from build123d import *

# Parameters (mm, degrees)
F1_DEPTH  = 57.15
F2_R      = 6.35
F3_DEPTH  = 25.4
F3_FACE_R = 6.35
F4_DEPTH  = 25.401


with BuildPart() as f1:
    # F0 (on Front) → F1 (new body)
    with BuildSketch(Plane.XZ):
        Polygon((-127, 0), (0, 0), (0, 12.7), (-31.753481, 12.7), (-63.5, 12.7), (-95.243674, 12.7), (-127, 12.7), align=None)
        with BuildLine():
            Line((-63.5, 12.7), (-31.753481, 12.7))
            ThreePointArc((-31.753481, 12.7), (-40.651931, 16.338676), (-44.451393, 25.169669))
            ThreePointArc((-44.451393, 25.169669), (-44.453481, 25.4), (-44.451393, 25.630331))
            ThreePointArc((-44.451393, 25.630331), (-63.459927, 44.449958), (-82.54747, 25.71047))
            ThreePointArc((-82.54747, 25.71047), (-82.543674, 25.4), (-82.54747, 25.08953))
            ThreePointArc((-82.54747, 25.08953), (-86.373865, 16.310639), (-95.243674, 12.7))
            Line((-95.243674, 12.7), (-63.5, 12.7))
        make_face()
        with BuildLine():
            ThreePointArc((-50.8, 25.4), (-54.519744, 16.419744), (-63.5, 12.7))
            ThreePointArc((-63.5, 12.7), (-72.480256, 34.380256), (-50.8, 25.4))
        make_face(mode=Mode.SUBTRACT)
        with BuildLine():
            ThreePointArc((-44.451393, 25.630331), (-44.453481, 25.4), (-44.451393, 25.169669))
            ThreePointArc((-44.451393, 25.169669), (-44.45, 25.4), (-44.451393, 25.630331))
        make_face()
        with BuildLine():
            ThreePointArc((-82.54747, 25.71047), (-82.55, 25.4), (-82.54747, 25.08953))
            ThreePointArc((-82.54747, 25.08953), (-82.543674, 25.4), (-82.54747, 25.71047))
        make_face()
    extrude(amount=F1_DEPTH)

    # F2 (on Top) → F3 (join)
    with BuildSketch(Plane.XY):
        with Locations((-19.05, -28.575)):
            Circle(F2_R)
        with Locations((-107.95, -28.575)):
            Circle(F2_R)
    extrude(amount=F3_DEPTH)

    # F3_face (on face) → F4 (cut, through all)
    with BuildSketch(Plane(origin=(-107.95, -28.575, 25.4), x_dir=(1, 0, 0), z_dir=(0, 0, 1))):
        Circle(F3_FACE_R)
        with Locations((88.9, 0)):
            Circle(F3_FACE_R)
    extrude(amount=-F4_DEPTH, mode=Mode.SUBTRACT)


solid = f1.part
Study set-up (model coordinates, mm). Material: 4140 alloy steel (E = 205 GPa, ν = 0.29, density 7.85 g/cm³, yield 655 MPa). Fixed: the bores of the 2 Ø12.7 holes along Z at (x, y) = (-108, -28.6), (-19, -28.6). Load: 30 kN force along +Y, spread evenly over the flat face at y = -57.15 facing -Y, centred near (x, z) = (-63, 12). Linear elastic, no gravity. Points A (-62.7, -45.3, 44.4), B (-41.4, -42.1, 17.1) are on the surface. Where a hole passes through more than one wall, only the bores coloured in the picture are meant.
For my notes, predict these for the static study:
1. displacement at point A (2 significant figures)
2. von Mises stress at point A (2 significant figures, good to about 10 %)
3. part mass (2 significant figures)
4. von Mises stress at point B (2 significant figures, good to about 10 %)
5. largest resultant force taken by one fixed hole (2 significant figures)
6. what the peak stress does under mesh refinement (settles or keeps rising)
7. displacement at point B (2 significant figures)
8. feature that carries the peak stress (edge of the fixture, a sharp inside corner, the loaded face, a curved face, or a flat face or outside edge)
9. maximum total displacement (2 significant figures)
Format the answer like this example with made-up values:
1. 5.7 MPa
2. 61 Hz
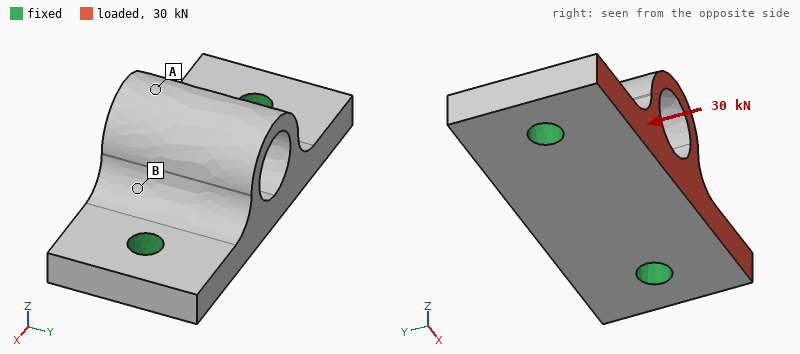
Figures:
1. 33 µm
2. 14 MPa
3. 970 g
4. 37 MPa
5. 15 kN
6. keeps rising
7. 14 µm
8. edge of the fixture
9. 37 µm
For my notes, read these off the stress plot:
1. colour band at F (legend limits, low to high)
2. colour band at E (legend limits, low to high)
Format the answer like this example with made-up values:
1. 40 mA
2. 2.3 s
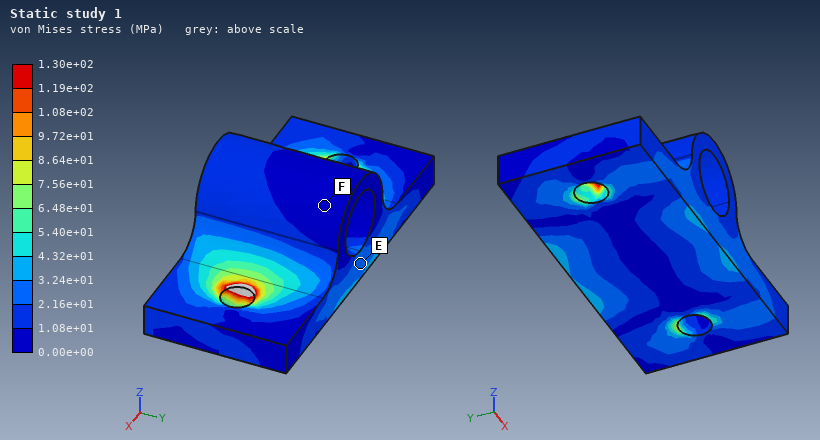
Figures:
1. 0.00e+00 to 1.08e+01 MPa
2. 2.16e+01 to 3.24e+01 MPa
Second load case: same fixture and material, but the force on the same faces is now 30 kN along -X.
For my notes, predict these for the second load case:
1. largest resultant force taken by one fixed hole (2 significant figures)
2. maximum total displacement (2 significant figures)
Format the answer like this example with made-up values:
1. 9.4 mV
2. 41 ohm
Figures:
1. 17 kN
2. 25 µm
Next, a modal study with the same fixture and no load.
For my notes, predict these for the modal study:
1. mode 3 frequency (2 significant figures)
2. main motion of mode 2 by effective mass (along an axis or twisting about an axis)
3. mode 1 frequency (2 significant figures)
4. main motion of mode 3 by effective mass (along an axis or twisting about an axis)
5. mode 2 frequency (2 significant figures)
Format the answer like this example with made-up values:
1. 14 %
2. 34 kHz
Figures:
1. 9800 Hz
2. along Z
3. 4700 Hz
4. along X
5. 6600 Hz
